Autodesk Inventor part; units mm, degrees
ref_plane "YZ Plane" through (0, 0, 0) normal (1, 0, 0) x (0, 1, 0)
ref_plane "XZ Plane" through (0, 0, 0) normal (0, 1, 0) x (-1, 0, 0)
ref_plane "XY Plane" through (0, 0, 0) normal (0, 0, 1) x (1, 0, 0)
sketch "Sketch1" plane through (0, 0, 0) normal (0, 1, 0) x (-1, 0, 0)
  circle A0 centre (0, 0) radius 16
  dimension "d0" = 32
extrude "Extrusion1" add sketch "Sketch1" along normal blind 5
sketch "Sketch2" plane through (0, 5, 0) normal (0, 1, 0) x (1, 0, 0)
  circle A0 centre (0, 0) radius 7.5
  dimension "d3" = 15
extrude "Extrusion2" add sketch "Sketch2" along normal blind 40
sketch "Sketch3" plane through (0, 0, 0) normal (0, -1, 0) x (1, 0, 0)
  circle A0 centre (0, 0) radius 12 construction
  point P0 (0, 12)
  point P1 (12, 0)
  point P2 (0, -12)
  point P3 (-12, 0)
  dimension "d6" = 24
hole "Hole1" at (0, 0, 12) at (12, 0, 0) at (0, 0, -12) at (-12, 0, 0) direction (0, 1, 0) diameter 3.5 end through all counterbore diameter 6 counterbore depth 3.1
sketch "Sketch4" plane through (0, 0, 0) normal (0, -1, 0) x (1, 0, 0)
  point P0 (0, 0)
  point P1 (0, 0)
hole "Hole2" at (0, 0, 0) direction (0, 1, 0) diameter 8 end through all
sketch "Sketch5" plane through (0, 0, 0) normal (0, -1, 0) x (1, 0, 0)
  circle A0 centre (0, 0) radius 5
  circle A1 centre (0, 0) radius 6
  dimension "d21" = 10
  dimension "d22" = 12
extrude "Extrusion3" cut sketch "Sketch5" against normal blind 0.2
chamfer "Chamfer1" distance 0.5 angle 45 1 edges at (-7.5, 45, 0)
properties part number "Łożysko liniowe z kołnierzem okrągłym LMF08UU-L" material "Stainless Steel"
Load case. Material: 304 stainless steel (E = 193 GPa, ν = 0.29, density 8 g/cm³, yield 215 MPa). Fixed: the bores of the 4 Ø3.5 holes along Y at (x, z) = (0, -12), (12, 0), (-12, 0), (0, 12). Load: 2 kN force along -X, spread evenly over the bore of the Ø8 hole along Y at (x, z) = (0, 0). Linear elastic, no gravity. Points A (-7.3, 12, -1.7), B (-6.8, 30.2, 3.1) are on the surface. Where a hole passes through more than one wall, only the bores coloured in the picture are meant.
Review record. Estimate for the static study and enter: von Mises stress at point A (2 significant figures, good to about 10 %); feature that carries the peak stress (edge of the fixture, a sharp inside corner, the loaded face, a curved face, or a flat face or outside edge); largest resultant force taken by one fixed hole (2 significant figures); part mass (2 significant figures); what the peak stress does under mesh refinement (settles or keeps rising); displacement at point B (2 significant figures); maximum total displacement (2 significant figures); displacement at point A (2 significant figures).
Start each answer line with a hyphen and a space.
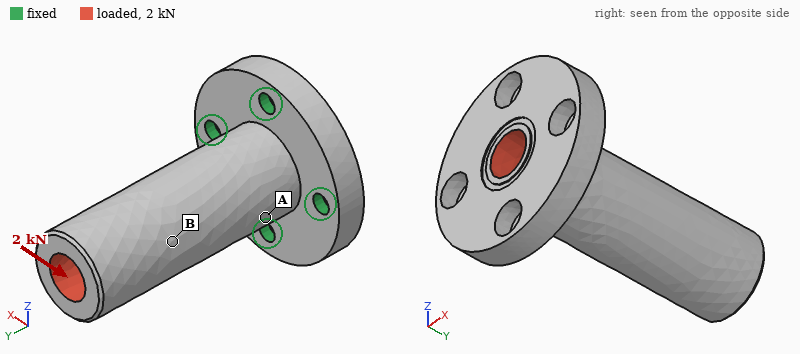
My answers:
- 74 MPa
- edge of the fixture
- 1.6 kN
- 67 g
- keeps rising
- 46 µm
- 74 µm
- 15 µm
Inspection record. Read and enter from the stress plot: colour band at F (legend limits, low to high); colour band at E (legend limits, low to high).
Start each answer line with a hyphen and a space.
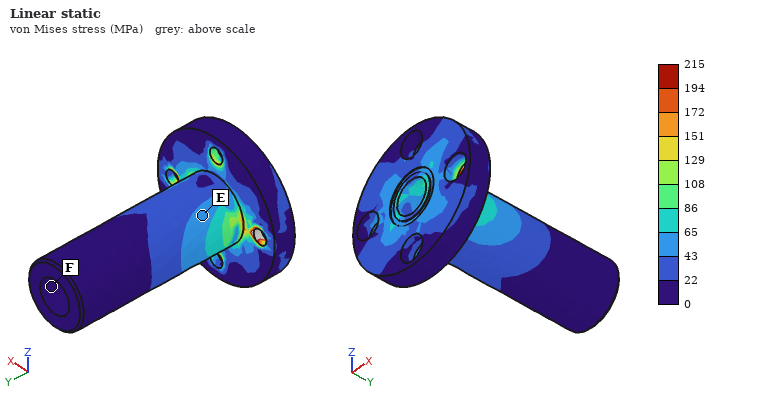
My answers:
- 0 to 22 MPa
- 43 to 65 MPa
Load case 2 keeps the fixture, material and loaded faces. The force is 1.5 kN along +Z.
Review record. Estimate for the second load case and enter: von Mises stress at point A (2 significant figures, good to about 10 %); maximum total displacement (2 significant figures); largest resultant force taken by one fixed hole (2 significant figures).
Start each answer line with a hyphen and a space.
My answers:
- 22 MPa
- 55 µm
- 1.2 kN
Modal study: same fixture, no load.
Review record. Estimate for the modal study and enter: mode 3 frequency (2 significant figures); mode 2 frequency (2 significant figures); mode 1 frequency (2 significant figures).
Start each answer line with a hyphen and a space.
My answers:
- 18 kHz
- 4700 Hz
- 4700 Hz
